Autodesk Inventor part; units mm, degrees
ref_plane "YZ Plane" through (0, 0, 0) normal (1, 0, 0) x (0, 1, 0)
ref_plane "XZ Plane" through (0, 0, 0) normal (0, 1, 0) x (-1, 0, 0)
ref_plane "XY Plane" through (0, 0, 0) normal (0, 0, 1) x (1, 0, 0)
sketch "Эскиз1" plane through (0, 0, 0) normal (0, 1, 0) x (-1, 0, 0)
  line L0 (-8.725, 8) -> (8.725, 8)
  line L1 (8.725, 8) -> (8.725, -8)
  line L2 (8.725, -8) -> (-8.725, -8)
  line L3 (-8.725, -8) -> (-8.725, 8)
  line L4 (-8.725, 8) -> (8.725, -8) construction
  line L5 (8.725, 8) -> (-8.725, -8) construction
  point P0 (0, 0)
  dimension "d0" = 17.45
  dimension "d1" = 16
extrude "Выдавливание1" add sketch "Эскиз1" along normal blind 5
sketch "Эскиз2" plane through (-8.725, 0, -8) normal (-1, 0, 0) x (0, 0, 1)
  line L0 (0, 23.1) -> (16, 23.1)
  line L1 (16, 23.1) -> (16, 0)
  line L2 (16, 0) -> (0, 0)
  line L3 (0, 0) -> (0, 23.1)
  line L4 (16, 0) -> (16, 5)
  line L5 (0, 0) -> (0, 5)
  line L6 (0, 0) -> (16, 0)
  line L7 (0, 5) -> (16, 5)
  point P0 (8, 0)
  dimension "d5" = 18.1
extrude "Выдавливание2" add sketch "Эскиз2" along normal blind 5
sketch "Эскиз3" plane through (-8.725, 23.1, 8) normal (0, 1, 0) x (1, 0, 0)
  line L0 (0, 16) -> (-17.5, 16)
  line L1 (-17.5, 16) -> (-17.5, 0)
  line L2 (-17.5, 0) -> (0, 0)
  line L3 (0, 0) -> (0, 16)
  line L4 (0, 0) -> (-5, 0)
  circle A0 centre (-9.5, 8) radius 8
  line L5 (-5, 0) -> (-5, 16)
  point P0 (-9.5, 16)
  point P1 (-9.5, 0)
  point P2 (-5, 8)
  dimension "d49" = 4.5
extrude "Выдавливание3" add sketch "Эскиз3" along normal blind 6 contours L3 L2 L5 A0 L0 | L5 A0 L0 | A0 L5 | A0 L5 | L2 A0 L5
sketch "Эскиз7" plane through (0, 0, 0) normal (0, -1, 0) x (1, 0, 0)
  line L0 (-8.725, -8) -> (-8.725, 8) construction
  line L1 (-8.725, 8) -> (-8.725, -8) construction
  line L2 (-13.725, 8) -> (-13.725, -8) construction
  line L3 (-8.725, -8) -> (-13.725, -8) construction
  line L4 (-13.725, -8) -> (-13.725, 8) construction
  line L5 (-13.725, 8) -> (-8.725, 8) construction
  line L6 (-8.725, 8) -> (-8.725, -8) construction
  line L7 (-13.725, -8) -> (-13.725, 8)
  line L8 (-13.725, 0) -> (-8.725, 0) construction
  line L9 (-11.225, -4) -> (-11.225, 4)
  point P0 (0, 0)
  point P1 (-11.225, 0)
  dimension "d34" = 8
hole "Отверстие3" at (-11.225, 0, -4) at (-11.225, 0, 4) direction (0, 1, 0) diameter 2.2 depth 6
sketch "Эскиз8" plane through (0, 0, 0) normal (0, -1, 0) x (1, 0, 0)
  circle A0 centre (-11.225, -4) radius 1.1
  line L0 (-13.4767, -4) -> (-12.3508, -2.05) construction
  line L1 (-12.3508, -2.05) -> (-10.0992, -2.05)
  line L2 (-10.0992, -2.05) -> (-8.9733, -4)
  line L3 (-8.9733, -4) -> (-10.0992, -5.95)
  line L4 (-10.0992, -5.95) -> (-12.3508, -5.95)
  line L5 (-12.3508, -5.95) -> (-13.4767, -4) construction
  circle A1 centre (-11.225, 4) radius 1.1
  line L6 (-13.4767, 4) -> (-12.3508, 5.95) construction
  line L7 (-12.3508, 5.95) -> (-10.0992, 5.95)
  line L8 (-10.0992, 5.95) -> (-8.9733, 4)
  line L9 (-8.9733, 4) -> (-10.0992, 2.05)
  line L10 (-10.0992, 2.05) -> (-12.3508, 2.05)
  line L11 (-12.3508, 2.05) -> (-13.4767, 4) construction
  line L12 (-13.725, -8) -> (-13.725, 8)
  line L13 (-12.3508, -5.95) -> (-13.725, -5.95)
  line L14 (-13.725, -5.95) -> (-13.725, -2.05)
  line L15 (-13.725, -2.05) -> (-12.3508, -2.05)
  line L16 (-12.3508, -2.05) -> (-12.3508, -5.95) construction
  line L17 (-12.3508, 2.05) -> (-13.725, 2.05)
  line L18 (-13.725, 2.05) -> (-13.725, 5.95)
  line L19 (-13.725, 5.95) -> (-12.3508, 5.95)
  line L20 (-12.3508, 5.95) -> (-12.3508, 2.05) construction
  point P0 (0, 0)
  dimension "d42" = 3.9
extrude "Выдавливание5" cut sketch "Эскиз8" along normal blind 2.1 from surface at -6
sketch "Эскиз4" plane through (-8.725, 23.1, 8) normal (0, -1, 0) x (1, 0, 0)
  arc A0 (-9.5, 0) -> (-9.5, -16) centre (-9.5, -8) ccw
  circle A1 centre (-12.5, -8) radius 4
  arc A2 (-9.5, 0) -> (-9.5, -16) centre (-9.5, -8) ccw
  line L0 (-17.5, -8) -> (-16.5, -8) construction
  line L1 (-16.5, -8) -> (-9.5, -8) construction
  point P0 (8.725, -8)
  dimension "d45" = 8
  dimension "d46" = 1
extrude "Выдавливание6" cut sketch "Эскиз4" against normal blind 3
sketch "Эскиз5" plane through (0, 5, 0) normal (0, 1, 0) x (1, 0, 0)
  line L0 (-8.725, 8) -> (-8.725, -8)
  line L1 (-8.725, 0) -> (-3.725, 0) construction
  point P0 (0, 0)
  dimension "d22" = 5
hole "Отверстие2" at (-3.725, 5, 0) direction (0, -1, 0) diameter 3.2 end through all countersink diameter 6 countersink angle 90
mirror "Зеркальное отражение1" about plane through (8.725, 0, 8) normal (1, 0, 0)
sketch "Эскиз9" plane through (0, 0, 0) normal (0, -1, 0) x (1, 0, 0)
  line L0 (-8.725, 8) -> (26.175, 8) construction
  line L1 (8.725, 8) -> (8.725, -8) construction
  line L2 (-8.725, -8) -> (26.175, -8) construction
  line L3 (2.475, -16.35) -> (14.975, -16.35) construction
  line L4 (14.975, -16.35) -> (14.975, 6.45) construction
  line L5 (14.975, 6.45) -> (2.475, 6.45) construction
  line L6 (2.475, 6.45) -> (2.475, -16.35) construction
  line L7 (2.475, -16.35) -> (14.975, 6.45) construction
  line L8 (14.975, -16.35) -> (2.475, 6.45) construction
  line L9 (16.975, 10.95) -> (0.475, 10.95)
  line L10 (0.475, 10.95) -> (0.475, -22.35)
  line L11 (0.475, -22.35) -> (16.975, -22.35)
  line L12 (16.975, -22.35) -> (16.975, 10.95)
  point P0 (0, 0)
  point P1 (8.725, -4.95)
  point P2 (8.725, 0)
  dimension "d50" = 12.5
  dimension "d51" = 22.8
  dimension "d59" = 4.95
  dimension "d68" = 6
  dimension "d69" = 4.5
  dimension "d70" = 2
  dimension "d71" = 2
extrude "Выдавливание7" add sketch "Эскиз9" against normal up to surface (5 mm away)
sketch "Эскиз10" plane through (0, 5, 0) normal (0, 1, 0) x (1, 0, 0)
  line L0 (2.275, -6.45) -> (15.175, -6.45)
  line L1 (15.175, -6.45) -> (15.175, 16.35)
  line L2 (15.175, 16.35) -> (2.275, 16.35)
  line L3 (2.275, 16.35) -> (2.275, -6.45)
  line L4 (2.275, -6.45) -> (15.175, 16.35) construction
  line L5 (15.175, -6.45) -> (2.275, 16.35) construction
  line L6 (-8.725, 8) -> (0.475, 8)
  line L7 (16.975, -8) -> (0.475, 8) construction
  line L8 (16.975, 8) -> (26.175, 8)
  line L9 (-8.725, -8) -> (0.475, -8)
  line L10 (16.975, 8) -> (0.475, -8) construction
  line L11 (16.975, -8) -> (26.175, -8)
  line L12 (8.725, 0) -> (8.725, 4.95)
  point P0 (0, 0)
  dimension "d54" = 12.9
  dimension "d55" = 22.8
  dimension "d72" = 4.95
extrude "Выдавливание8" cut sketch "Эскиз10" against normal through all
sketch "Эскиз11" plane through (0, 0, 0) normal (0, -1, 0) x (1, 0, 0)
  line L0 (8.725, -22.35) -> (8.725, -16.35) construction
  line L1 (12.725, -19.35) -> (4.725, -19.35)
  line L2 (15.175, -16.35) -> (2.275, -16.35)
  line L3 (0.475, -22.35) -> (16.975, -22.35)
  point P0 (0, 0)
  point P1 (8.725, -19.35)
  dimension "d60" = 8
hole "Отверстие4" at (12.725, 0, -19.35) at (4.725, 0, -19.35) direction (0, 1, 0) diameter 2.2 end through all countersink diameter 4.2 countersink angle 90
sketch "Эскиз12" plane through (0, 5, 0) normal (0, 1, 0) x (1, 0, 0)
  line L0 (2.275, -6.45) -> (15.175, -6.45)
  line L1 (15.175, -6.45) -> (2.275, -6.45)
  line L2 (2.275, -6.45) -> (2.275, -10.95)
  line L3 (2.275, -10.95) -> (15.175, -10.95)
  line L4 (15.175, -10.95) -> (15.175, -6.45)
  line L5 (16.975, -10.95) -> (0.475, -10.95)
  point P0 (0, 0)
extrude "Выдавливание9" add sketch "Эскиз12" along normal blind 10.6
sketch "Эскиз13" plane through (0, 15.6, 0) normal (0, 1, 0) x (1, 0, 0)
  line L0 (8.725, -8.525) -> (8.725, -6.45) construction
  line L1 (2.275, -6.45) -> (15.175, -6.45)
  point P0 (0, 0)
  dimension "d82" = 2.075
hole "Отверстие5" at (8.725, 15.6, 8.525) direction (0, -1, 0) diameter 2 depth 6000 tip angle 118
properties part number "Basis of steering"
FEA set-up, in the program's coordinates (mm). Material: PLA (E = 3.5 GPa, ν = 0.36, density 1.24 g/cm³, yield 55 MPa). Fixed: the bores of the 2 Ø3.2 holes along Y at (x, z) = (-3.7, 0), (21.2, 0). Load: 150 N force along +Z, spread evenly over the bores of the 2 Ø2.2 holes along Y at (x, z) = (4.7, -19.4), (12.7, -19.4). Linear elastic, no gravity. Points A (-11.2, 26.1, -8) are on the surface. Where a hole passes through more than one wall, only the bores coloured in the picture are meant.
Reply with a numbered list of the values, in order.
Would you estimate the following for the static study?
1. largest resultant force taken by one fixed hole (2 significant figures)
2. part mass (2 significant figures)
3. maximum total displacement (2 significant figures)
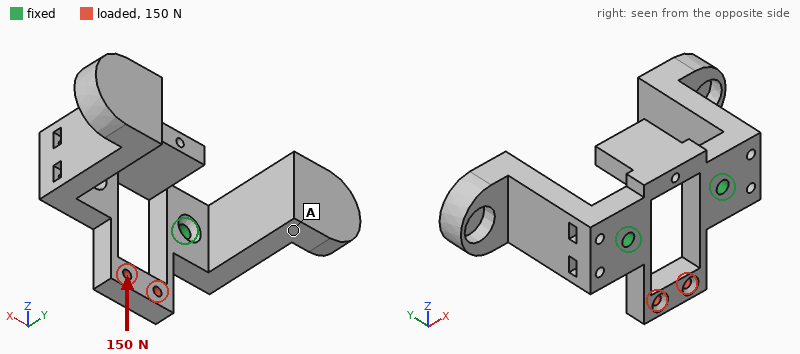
1. 76 N
2. 12 g
3. 0.14 mm
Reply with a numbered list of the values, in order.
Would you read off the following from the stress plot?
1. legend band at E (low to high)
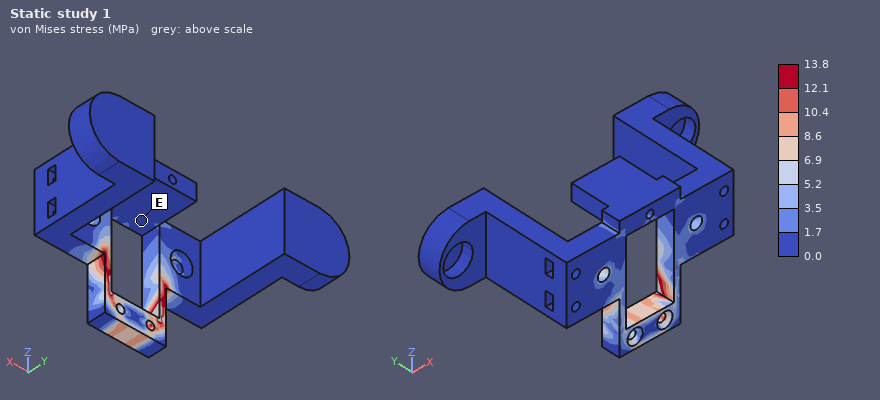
1. 0.0 to 1.7 MPa
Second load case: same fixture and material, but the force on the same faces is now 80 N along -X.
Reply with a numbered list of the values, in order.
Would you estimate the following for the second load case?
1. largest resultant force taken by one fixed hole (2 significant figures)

1. 58 N
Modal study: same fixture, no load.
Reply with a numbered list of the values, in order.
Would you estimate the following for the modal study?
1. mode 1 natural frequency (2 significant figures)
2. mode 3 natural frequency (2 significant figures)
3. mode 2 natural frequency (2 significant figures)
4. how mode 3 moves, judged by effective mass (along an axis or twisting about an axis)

1. 760 Hz
2. 1100 Hz
3. 760 Hz
4. along Z
